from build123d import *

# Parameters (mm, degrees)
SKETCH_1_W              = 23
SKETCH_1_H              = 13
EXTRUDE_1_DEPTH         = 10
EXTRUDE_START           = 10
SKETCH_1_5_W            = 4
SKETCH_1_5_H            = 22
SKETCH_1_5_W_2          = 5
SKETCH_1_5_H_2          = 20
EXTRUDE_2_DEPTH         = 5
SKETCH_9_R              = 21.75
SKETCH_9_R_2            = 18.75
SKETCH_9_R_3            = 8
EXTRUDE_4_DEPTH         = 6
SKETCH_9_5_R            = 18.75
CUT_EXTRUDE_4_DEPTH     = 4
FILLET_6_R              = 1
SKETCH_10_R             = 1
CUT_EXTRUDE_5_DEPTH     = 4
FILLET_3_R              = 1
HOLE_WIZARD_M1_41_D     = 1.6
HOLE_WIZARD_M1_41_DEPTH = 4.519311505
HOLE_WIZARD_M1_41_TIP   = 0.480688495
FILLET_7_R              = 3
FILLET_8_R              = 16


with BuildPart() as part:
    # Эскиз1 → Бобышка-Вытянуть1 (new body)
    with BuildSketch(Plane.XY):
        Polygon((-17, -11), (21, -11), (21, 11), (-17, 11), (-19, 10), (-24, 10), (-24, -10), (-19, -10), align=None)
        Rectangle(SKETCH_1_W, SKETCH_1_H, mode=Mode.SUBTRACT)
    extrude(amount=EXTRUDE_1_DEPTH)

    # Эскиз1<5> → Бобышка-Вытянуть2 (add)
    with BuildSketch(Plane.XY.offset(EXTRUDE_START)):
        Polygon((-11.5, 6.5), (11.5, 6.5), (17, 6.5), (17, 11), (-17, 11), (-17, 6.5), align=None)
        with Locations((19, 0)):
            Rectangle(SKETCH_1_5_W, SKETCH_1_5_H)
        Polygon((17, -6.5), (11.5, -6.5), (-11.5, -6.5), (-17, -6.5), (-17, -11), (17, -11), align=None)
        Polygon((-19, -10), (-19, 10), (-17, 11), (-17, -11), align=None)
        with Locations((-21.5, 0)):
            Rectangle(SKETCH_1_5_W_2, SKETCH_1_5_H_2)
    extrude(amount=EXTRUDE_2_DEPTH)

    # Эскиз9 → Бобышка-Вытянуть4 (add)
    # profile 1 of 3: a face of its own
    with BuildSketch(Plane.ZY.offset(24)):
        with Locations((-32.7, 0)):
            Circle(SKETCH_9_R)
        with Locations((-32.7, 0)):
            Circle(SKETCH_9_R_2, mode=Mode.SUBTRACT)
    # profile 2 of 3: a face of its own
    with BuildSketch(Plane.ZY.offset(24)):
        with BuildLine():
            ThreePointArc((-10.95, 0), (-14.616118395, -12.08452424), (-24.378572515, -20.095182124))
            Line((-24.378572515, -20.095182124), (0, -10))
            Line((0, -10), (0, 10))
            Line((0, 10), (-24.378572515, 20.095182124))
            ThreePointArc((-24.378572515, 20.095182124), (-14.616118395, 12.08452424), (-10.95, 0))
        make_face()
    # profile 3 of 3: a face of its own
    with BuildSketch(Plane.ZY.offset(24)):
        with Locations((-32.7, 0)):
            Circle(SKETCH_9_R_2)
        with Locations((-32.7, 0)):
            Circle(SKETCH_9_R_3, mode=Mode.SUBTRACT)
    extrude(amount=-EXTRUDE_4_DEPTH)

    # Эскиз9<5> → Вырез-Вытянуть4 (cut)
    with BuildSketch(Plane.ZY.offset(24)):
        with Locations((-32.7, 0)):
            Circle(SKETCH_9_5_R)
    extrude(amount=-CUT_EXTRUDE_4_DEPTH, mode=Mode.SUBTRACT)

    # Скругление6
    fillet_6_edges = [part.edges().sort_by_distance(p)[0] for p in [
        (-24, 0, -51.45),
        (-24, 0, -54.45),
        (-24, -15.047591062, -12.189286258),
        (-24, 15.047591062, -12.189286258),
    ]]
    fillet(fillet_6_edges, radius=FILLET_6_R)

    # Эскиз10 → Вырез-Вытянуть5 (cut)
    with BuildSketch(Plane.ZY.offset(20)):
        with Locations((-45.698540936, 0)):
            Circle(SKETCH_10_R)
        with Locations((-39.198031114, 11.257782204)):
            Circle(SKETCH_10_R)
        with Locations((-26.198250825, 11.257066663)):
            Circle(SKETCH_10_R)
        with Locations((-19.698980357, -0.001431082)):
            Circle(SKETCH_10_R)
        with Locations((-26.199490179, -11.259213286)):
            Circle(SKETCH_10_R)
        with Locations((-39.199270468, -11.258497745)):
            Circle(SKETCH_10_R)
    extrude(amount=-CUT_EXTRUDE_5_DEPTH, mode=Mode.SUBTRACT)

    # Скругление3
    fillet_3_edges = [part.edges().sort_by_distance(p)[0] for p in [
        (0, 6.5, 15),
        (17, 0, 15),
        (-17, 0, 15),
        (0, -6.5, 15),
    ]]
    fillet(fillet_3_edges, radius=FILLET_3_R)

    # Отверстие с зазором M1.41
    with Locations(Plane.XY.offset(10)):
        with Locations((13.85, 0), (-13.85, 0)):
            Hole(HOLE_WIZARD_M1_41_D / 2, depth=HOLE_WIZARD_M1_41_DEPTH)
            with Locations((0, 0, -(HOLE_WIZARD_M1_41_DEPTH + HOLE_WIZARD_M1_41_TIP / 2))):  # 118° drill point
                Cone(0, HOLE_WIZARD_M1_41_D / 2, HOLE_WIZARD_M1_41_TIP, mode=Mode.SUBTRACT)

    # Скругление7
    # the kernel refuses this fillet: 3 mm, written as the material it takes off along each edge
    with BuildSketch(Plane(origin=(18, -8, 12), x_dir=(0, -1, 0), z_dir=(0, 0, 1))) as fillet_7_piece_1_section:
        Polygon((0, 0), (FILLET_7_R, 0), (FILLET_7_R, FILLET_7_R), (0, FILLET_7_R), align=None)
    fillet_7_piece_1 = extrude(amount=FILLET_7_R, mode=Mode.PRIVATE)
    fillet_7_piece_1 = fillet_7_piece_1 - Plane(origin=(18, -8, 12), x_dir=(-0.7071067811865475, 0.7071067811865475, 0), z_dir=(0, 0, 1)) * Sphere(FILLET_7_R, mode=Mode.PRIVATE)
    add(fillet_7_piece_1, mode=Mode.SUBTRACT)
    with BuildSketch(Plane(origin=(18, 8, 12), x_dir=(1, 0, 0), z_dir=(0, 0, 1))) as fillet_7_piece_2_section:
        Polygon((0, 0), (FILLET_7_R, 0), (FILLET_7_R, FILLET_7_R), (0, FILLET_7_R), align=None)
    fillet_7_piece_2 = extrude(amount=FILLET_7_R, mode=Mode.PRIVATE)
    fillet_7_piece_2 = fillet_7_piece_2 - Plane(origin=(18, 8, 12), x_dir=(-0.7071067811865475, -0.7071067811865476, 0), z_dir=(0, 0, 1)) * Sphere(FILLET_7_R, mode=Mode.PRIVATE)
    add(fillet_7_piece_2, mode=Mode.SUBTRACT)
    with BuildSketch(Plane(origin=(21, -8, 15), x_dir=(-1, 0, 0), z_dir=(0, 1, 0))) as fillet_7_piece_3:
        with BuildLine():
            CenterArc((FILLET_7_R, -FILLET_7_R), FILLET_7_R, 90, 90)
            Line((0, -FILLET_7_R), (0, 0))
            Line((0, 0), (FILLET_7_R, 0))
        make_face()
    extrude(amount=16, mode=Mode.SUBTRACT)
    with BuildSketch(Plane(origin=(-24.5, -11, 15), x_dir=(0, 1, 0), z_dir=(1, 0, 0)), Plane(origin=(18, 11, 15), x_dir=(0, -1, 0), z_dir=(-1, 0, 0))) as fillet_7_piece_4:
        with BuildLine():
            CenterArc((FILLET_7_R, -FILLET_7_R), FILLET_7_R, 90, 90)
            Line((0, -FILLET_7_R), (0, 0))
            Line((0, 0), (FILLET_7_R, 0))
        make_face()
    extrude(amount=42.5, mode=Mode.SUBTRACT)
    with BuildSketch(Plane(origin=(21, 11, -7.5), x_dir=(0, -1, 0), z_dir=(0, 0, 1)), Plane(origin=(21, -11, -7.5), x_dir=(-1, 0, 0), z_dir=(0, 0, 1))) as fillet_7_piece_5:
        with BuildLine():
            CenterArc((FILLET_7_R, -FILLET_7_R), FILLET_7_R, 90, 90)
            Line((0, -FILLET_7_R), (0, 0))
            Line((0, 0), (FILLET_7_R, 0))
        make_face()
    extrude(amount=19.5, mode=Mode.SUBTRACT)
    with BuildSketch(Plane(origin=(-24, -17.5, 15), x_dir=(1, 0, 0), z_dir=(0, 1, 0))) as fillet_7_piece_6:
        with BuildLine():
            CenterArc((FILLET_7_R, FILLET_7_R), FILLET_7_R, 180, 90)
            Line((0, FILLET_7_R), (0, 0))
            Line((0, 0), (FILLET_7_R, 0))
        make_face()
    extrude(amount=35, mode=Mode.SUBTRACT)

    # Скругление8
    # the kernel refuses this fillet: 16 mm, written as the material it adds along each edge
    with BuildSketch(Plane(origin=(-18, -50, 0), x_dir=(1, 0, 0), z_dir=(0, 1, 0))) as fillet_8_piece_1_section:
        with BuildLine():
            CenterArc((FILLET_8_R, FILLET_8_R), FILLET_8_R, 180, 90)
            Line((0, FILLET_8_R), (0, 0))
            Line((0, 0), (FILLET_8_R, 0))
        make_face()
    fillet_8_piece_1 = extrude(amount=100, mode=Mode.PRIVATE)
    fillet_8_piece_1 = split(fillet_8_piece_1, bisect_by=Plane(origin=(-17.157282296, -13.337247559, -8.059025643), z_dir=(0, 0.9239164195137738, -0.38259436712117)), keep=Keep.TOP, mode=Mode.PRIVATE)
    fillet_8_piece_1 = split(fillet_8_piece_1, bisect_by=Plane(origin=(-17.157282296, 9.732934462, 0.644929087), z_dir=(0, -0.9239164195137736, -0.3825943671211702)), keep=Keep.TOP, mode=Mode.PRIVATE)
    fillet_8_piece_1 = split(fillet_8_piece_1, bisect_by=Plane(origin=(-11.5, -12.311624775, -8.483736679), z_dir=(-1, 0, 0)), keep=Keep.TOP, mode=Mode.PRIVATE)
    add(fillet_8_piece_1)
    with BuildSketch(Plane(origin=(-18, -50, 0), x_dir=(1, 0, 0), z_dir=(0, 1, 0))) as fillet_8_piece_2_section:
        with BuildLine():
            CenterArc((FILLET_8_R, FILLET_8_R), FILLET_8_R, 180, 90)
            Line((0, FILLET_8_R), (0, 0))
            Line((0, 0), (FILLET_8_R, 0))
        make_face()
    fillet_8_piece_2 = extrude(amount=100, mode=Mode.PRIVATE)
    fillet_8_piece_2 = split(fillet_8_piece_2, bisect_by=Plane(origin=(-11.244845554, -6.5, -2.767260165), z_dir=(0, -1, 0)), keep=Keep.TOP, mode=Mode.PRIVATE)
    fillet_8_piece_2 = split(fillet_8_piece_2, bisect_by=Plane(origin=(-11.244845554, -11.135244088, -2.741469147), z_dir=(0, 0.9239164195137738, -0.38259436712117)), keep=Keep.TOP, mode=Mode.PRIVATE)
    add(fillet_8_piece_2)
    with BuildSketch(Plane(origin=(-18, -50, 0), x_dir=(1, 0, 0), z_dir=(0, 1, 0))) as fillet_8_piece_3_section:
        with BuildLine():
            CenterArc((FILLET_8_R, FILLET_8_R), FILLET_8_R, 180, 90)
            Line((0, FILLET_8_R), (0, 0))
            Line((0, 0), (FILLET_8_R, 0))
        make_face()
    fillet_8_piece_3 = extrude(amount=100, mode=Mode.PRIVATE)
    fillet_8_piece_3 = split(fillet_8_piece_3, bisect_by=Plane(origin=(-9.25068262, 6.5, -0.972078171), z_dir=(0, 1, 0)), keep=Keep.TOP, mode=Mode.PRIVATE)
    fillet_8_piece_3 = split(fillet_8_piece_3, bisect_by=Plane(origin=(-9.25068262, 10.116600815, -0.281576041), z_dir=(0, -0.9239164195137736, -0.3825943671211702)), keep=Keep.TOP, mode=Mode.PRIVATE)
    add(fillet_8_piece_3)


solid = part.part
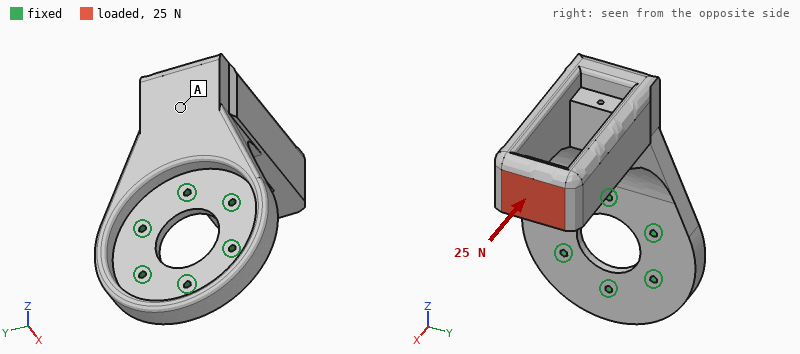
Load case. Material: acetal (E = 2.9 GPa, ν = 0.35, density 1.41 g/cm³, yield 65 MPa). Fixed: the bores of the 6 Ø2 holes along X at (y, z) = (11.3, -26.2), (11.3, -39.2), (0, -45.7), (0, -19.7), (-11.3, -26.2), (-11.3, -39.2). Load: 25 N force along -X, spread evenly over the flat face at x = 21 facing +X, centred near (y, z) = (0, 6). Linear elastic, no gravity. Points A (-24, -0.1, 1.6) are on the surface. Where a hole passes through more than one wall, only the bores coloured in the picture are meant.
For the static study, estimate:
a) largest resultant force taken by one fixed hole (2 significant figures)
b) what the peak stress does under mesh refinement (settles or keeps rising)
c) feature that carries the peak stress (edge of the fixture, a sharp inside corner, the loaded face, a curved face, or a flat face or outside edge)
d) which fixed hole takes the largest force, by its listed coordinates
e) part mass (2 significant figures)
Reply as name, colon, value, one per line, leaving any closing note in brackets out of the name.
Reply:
largest resultant force taken by one fixed hole: 59 N
what the peak stress does under mesh refinement: keeps rising
feature that carries the peak stress: edge of the fixture
which fixed hole takes the largest force, by its listed coordinates: (0, -19.7)
part mass: 23 g
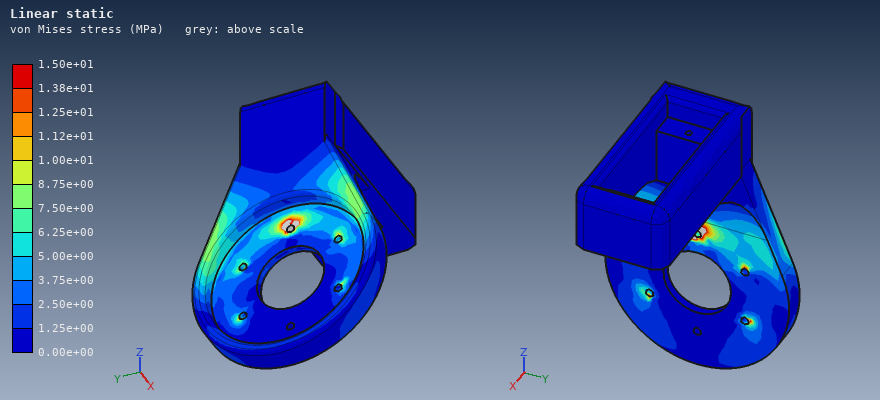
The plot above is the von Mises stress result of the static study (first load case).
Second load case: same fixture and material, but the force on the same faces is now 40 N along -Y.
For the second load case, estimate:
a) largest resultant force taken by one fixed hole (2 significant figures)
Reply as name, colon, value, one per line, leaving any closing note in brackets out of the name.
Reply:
largest resultant force taken by one fixed hole: 64 N
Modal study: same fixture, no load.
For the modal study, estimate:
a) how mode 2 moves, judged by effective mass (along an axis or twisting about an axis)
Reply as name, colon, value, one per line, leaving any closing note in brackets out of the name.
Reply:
how mode 2 moves, judged by effective mass: along Y
